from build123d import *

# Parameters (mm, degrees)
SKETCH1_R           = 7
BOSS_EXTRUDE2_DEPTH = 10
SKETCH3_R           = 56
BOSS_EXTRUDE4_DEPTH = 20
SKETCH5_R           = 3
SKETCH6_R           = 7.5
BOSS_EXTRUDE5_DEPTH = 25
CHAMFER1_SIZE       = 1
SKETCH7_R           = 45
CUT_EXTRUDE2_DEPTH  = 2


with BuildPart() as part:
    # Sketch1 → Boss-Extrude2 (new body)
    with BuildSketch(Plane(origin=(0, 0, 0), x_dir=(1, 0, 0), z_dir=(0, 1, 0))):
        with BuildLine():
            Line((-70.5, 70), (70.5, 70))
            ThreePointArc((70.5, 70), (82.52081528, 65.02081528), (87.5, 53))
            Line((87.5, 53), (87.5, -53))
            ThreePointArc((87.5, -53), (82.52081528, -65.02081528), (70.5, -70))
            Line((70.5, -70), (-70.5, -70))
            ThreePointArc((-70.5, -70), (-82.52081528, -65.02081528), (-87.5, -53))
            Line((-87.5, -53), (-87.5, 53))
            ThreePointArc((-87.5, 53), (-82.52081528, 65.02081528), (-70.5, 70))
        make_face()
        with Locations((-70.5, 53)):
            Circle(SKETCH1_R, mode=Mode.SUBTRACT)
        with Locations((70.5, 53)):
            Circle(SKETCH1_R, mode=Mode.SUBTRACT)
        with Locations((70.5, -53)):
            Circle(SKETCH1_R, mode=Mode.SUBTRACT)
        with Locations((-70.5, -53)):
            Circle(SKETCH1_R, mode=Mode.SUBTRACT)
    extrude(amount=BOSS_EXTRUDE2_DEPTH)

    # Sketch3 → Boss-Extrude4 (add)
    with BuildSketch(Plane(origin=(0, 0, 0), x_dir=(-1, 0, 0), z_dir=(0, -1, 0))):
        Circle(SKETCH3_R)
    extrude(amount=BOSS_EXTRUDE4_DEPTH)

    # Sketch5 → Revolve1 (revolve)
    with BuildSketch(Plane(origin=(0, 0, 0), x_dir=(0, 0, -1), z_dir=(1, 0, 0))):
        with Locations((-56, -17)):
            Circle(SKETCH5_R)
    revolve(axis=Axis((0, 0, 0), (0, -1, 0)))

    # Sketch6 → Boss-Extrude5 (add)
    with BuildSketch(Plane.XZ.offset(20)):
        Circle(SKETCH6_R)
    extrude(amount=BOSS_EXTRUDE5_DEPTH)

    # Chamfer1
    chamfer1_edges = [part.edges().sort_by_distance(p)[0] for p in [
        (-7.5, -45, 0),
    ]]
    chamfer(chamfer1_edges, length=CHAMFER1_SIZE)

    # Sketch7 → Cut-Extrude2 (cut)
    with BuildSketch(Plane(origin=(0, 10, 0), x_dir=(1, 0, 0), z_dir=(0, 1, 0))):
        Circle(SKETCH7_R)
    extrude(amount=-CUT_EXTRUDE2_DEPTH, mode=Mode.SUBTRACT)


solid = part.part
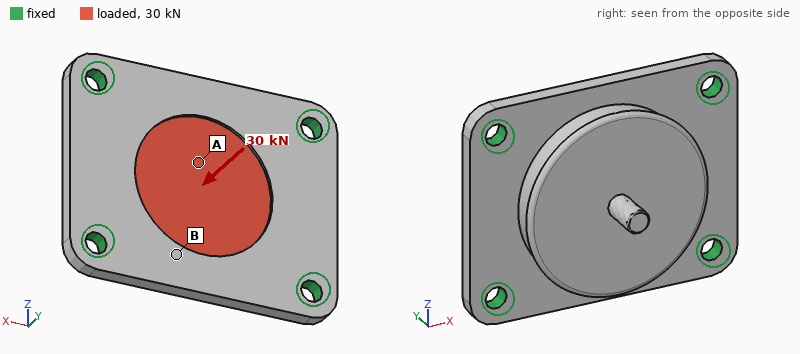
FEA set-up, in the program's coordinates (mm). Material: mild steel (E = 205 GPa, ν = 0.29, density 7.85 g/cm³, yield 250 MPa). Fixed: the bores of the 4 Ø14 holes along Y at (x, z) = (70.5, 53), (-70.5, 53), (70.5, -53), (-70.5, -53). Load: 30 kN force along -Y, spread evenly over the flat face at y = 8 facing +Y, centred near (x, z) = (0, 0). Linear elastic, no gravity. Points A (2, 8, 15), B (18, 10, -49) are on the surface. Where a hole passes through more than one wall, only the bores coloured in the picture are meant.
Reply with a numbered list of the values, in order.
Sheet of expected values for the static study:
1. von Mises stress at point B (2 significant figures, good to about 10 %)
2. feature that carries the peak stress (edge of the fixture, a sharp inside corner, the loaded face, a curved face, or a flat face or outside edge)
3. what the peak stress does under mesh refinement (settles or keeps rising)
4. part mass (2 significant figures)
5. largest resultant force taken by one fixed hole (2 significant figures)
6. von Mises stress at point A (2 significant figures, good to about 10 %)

1. 31 MPa
2. edge of the fixture
3. keeps rising
4. 3.4 kg
5. 9.2 kN
6. 18 MPa
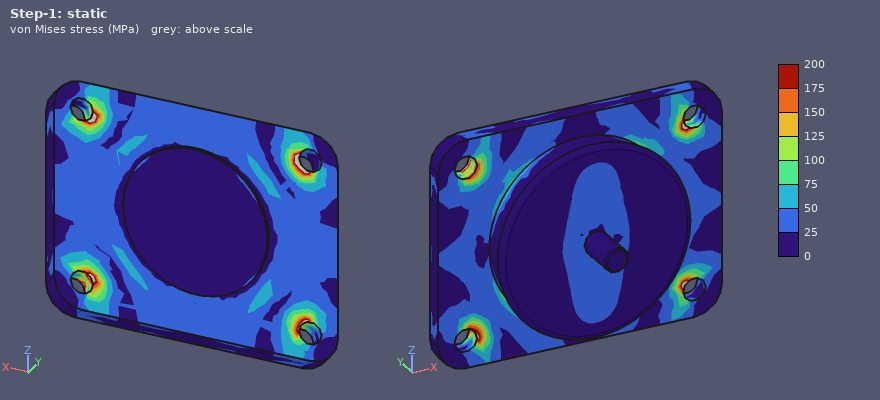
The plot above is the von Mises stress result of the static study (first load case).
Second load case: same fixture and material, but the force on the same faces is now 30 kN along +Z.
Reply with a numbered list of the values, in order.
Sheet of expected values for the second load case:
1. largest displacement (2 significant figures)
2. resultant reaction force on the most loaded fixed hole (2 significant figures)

1. 12 µm
2. 8.2 kN
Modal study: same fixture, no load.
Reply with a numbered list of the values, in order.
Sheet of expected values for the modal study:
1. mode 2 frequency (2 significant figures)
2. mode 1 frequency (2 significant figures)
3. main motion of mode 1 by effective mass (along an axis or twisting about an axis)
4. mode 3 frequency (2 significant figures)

1. 3300 Hz
2. 2600 Hz
3. along Y
4. 4500 Hz
